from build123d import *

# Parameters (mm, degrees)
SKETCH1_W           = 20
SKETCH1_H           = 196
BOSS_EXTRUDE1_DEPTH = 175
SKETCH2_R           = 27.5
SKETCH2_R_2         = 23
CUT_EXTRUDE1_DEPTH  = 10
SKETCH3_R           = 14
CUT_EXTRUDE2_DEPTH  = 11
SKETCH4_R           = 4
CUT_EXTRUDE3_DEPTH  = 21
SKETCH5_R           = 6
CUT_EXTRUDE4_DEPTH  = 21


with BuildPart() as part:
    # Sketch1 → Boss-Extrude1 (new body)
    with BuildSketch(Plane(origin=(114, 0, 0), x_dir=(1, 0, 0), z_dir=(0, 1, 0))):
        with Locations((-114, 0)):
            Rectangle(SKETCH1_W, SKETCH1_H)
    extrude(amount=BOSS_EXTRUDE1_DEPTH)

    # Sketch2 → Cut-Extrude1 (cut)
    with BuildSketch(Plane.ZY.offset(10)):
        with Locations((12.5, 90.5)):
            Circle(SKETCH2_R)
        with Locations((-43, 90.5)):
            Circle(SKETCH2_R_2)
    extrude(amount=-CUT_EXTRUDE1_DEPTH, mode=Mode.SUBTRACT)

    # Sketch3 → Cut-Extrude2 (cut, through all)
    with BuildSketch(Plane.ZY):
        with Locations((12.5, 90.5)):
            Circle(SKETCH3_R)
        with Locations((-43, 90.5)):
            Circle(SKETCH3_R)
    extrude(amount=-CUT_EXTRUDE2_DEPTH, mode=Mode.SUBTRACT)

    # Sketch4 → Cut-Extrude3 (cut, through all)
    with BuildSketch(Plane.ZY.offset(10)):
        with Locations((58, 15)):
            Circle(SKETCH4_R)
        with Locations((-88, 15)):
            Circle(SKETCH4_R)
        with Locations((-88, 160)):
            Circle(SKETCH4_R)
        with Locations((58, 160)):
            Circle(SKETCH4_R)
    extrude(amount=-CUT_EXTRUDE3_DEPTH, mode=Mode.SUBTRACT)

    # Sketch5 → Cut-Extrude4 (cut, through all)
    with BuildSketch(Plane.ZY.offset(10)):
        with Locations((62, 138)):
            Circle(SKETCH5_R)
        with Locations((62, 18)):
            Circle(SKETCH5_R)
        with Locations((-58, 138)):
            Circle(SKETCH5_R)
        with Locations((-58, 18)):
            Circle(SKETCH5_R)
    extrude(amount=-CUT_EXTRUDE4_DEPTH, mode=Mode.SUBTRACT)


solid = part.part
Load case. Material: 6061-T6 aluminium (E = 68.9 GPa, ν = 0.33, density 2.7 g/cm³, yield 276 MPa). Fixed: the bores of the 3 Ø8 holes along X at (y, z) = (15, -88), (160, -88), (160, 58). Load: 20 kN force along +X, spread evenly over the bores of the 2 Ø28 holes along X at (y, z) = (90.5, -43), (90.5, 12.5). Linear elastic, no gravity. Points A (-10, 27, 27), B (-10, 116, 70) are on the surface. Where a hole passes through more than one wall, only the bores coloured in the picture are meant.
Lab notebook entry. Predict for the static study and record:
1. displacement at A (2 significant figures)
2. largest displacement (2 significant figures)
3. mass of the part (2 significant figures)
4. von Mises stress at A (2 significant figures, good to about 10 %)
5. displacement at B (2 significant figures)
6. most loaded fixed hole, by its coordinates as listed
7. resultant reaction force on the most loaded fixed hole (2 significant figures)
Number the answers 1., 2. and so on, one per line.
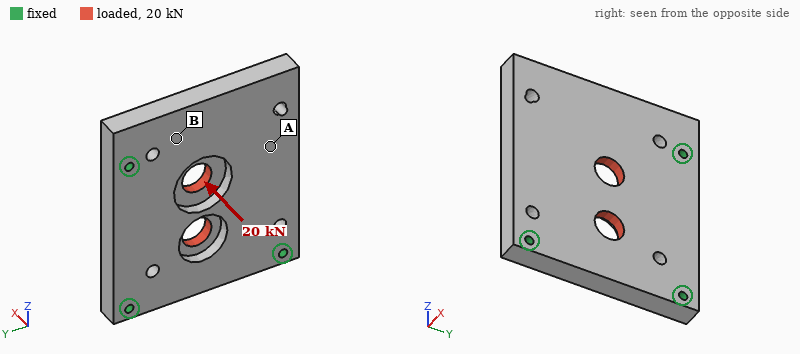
1. 0.29 mm
2. 0.37 mm
3. 1.7 kg
4. 37 MPa
5. 0.12 mm
6. (160, 58)
7. 8.9 kN
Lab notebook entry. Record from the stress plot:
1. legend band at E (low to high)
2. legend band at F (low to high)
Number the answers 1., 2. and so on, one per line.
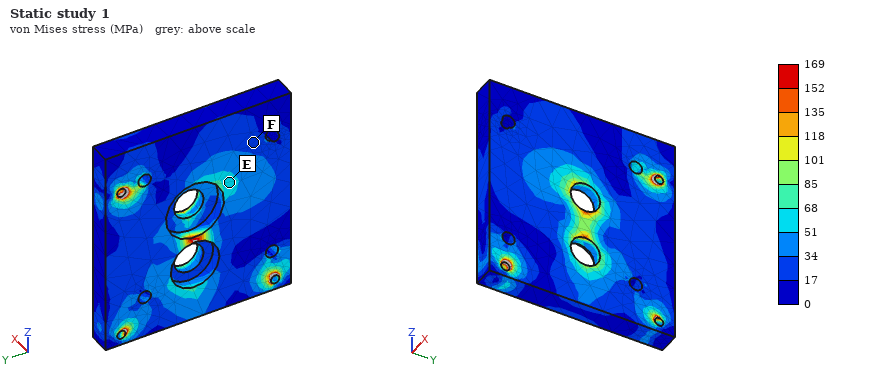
1. 51 to 68 MPa
2. 17 to 34 MPa
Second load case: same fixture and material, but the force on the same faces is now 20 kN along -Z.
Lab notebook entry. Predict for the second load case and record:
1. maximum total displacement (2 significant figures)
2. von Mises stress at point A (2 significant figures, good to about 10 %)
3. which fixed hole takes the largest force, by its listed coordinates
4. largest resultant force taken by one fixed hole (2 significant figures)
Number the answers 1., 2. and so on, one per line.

1. 44 µm
2. 4.5 MPa
3. (15, -88)
4. 8.2 kN
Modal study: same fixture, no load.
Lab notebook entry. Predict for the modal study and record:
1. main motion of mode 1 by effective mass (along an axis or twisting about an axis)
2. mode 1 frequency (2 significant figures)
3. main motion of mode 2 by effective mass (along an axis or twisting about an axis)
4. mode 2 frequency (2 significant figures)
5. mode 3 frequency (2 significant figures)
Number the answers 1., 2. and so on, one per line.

1. along X
2. 870 Hz
3. along X
4. 2600 Hz
5. 3100 Hz
